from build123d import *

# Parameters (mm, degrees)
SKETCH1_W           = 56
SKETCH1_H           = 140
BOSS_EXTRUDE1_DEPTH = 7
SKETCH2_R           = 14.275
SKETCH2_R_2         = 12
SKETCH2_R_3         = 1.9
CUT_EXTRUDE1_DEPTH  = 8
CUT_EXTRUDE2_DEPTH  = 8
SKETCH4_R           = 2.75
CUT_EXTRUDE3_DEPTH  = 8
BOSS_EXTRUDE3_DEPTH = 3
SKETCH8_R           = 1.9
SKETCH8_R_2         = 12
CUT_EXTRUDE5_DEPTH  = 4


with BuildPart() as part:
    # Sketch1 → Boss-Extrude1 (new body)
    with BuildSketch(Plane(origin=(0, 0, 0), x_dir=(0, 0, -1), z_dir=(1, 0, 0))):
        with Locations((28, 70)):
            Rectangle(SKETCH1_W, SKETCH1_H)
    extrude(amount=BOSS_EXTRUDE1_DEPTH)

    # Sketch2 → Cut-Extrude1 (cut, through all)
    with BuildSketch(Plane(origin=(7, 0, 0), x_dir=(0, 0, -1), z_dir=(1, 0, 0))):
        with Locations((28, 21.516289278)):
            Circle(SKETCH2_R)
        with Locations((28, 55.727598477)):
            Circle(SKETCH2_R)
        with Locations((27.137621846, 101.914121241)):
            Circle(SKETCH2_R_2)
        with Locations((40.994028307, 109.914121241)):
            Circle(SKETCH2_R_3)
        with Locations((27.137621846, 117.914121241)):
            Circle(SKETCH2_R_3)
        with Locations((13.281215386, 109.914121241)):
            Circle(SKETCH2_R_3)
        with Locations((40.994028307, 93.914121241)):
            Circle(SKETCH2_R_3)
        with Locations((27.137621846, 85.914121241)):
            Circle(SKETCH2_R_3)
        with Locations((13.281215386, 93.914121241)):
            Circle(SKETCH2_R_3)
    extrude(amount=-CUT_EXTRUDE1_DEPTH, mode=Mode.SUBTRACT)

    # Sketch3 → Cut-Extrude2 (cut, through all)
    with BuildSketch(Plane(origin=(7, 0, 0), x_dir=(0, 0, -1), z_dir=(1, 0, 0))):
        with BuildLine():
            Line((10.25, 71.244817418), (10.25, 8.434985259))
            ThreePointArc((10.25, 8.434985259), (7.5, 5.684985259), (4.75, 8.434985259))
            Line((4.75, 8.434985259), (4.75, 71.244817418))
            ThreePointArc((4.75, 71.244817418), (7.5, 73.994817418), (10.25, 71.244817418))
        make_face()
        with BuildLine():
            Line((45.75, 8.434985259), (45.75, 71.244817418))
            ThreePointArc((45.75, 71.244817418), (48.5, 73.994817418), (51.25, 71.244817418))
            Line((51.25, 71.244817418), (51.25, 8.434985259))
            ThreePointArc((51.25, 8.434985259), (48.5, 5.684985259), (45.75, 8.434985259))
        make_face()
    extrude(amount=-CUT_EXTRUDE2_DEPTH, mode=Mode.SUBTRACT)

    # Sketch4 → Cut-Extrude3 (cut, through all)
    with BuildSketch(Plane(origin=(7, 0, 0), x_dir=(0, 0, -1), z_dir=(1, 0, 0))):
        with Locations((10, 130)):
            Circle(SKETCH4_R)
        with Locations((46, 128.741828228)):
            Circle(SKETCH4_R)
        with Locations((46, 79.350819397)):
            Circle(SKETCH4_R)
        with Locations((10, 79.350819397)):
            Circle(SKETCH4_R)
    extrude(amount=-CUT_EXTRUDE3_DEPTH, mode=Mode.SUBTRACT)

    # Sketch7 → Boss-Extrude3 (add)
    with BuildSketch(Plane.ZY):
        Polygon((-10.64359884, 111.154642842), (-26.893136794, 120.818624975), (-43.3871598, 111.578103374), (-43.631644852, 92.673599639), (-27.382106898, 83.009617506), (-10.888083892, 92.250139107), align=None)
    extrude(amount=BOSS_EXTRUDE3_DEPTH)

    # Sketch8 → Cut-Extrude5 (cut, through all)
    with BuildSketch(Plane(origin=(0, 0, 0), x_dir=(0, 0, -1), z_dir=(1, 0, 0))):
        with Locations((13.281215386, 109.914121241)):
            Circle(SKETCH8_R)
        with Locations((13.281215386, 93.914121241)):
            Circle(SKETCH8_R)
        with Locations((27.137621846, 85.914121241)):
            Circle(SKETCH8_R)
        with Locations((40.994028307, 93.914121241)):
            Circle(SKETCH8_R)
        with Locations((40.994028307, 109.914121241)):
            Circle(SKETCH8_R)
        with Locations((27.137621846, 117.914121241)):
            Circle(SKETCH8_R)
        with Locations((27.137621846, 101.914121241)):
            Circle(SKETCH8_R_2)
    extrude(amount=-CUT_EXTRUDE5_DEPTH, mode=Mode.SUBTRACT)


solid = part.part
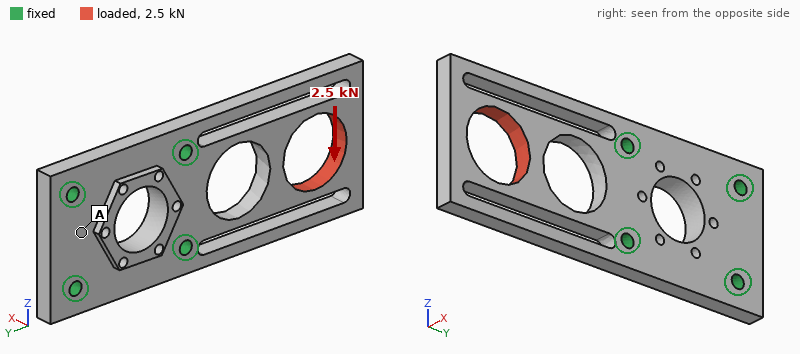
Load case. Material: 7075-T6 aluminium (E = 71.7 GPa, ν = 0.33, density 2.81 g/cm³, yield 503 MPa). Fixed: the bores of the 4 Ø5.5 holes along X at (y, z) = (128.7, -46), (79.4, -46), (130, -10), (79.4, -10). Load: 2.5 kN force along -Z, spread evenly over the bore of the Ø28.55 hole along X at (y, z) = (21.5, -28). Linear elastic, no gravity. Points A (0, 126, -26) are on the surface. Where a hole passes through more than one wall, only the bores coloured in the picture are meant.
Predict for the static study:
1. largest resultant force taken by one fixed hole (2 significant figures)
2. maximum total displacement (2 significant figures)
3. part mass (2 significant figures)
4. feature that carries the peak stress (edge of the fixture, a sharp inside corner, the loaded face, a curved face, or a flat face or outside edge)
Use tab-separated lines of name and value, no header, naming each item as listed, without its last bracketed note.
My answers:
largest resultant force taken by one fixed hole	3.7 kN
maximum total displacement	0.54 mm
part mass	110 g
feature that carries the peak stress	a flat face or outside edge
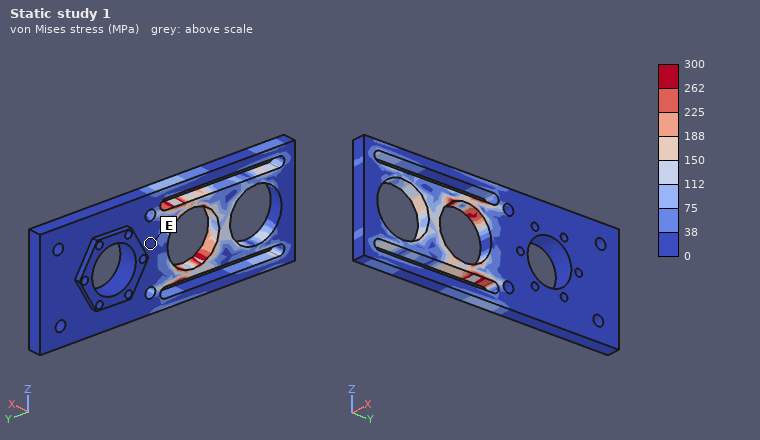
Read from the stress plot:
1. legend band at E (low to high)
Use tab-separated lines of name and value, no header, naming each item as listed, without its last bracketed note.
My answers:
legend band at E	0 to 38 MPa
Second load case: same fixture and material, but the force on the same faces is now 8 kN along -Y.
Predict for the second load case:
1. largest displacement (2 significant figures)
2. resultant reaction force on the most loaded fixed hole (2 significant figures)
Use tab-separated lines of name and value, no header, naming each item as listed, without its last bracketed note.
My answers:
largest displacement	0.13 mm
resultant reaction force on the most loaded fixed hole	3.8 kN
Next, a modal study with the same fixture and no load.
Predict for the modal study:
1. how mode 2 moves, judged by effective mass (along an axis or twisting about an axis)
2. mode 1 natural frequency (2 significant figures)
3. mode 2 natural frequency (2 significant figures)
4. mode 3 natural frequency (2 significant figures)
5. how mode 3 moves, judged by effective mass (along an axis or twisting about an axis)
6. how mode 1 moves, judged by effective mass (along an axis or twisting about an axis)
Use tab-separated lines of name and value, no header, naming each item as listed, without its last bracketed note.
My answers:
how mode 2 moves, judged by effective mass	twisting about Y
mode 1 natural frequency	750 Hz
mode 2 natural frequency	1800 Hz
mode 3 natural frequency	2100 Hz
how mode 3 moves, judged by effective mass	along Z
how mode 1 moves, judged by effective mass	along X
